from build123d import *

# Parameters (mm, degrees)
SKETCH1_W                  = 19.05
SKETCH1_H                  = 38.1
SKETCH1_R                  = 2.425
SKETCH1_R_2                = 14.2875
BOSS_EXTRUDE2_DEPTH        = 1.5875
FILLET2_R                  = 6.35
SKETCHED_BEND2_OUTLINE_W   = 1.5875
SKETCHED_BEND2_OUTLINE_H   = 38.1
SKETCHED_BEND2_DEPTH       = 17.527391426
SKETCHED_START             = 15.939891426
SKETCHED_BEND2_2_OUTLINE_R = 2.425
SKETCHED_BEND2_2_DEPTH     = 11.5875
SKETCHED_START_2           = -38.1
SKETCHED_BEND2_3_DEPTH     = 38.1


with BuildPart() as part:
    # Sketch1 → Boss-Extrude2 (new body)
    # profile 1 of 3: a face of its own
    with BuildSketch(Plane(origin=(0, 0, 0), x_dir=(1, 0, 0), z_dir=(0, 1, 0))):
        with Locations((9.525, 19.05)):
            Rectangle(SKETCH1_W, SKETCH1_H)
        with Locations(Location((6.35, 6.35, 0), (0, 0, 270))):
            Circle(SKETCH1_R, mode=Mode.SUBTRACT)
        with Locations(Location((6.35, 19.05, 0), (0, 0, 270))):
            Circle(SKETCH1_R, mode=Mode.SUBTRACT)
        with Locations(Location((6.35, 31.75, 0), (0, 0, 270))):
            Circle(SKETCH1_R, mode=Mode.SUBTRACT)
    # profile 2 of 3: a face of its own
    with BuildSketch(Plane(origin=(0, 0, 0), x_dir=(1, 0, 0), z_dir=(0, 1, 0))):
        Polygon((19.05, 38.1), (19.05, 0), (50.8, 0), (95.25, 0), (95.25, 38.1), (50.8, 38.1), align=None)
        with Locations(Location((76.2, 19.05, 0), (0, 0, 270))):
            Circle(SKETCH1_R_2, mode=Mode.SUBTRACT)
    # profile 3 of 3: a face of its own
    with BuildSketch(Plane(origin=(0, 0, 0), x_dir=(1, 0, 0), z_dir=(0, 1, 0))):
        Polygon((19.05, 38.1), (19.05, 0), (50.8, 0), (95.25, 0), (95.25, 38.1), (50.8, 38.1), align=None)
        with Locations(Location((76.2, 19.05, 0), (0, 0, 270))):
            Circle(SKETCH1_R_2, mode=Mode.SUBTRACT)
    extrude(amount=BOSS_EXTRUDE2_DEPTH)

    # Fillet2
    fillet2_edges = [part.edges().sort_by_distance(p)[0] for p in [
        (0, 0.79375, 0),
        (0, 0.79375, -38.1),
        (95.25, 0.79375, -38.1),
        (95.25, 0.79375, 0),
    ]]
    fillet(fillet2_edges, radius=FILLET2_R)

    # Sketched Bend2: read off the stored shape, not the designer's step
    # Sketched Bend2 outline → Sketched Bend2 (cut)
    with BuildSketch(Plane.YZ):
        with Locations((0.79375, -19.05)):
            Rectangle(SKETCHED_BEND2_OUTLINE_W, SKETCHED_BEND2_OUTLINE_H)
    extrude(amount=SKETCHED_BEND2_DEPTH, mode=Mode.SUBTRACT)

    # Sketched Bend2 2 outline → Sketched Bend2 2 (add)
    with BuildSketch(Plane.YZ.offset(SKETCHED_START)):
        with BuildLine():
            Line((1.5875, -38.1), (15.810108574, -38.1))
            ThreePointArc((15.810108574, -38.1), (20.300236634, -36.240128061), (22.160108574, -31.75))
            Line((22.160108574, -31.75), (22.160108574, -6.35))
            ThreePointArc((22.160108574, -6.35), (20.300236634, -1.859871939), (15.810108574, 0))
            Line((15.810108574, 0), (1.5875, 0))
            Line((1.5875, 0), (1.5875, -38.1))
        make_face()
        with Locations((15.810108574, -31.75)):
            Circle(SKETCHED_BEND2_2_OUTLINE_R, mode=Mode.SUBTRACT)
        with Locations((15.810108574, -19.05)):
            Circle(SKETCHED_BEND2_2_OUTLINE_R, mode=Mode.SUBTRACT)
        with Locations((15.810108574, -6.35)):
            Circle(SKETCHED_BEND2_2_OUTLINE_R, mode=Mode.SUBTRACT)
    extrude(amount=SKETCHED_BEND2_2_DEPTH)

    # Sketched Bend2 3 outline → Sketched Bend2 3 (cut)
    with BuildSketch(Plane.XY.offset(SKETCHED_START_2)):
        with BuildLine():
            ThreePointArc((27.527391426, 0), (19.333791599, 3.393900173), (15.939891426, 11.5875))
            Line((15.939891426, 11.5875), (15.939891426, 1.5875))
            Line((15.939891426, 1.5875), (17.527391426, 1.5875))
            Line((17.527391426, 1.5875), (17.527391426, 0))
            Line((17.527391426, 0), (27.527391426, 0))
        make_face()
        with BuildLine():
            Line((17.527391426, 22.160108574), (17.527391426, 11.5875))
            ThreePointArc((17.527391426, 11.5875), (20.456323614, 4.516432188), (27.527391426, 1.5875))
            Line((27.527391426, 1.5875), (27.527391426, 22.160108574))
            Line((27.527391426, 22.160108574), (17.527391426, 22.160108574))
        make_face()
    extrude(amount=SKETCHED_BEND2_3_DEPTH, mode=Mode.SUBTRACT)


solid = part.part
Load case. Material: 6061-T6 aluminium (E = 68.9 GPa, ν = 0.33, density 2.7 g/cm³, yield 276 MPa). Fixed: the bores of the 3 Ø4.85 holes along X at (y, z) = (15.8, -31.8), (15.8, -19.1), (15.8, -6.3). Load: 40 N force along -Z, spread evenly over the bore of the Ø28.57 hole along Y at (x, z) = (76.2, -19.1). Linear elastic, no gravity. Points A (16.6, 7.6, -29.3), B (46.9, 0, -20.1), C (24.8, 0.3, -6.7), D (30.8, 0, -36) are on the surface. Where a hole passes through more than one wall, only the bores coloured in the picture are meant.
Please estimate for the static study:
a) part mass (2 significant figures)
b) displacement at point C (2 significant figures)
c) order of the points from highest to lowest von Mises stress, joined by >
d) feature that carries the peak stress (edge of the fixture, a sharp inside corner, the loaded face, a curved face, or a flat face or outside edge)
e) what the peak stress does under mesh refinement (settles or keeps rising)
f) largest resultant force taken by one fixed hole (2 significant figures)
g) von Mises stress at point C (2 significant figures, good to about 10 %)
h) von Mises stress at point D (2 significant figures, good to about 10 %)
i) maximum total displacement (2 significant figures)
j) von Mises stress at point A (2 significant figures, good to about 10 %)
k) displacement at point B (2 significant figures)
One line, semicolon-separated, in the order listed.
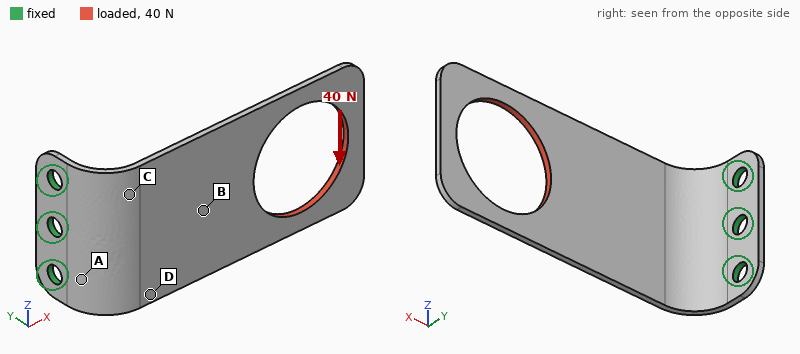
12 g; 0.093 mm; A > C > D > B; edge of the fixture; keeps rising; 91 N; 32 MPa; 21 MPa; 0.49 mm; 42 MPa; 0.15 mm
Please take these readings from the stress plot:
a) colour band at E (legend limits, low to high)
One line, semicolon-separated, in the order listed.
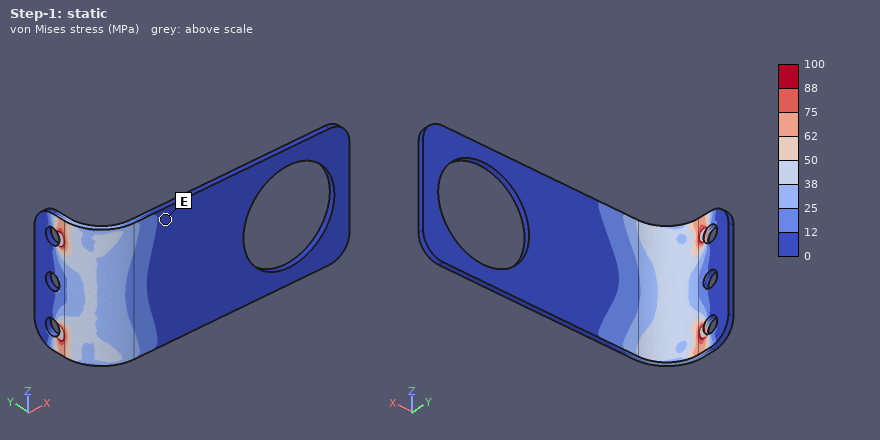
0 to 12 MPa
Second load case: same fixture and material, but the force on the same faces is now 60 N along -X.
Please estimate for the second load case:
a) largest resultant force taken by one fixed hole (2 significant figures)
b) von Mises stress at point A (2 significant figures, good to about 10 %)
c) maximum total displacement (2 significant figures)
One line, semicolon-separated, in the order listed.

20 N; 23 MPa; 0.48 mm
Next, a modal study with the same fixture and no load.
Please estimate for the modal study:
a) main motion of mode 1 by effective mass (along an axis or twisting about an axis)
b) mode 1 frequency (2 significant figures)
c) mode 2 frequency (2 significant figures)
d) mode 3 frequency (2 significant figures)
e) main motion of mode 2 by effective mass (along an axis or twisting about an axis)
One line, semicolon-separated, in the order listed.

along Y; 230 Hz; 710 Hz; 990 Hz; along Z
